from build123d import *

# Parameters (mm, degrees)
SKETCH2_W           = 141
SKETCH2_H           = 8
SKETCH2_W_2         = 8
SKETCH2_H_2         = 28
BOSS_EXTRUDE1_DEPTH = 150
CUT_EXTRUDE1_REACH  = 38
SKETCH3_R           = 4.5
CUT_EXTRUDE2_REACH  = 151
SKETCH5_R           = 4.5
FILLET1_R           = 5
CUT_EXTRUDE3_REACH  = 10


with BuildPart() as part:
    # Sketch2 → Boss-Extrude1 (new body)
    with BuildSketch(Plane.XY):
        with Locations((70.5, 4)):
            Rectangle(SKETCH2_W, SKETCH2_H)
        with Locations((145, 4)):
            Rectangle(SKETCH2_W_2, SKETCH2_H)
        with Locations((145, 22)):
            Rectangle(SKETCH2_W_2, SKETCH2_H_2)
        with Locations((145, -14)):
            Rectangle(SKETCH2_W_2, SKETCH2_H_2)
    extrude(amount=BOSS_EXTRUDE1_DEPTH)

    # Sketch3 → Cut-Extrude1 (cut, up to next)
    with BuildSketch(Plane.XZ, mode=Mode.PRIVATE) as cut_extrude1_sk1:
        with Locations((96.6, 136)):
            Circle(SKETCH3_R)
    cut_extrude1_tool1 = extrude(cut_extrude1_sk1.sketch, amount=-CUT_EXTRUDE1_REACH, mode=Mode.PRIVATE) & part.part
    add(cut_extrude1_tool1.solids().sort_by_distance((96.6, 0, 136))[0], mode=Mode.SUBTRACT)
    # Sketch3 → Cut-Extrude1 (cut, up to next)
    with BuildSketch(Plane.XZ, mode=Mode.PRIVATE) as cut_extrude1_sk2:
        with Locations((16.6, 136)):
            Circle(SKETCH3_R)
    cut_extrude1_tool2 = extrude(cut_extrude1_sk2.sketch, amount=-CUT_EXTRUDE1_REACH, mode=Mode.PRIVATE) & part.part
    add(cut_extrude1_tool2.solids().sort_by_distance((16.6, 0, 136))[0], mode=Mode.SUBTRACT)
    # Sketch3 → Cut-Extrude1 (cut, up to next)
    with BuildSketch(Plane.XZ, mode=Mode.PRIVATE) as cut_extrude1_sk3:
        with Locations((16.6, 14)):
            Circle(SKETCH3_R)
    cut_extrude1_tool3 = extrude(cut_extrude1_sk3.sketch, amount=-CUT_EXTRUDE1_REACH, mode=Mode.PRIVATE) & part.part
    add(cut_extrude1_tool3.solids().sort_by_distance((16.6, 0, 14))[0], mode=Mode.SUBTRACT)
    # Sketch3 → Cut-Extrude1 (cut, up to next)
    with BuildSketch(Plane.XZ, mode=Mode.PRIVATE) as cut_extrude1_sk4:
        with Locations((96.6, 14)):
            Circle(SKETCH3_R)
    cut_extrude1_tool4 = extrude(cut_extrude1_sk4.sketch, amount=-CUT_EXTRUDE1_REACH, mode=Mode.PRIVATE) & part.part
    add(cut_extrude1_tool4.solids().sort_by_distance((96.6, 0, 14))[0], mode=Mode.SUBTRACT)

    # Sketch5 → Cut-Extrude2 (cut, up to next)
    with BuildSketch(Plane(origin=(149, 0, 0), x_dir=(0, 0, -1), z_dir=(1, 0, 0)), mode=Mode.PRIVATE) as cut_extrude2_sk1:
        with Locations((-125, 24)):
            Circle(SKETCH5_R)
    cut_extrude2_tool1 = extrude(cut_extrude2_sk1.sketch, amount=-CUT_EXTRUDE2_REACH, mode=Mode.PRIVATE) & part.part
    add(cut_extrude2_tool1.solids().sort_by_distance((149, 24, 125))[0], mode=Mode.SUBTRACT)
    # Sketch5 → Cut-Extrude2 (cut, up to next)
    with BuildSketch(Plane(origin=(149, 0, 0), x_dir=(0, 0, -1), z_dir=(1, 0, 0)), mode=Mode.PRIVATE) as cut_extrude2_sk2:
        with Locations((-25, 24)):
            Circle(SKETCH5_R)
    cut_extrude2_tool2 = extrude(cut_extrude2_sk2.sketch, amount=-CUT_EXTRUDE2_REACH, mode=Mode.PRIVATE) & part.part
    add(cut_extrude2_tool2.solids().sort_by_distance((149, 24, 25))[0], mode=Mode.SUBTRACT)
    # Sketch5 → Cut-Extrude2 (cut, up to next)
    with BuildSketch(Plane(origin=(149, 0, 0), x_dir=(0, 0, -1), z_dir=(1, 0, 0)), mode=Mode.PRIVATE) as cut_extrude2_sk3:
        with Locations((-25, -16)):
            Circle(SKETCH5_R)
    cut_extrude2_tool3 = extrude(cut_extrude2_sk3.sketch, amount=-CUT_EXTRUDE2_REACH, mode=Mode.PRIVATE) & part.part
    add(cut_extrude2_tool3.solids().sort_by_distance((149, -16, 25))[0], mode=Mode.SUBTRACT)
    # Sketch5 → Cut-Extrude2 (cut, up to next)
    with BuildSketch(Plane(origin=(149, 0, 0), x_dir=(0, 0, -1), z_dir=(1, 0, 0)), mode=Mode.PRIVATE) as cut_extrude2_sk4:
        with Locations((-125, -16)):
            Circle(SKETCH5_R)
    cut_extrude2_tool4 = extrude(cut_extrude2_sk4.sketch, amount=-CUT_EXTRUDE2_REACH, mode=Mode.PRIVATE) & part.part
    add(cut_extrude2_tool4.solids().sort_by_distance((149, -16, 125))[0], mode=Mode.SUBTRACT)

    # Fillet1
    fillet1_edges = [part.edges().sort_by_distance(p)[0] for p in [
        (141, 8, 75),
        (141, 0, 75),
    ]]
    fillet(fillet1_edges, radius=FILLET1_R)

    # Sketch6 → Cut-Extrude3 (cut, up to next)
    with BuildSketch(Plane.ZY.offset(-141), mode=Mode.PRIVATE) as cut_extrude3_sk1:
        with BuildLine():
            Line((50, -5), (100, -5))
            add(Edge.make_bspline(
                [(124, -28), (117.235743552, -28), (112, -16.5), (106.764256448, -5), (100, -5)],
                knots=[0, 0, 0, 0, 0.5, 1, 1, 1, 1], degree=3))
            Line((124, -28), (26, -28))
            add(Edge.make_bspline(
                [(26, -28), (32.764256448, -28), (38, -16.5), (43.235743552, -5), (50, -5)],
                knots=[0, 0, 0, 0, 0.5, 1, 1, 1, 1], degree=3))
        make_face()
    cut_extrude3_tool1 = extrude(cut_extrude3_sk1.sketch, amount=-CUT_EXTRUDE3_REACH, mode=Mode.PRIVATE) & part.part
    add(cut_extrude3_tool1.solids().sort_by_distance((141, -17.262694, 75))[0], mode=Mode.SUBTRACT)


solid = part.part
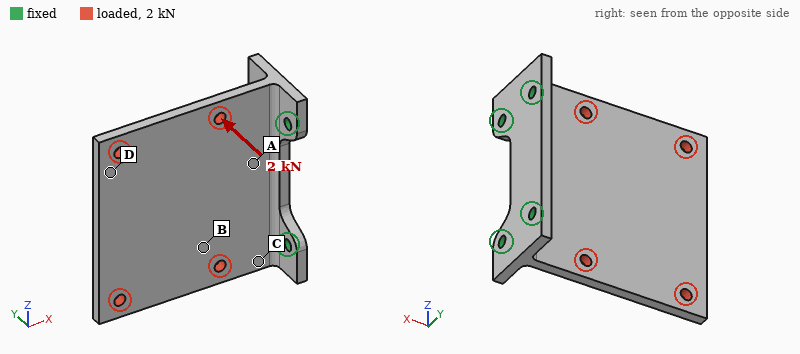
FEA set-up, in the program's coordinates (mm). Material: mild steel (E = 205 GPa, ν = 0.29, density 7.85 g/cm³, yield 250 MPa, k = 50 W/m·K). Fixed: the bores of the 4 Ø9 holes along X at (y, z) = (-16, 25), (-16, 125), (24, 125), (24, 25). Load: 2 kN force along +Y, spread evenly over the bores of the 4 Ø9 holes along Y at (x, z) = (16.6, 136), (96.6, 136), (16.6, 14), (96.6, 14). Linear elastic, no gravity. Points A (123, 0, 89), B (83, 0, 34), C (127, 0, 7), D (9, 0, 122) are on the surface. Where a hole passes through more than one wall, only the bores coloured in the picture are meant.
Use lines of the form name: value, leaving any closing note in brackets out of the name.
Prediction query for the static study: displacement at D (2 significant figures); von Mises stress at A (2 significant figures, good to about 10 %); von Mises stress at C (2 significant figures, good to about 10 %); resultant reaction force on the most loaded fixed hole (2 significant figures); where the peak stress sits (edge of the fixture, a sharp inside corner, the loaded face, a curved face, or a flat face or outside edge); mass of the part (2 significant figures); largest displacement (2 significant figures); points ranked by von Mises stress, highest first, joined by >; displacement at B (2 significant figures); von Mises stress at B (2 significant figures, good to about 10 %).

displacement at D: 0.66 mm
von Mises stress at A: 68 MPa
von Mises stress at C: 93 MPa
resultant reaction force on the most loaded fixed hole: 2.8 kN
where the peak stress sits: a curved face
mass of the part: 1.8 kg
largest displacement: 0.74 mm
points ranked by von Mises stress, highest first, joined by >: C > A > B > D
displacement at B: 0.19 mm
von Mises stress at B: 39 MPa
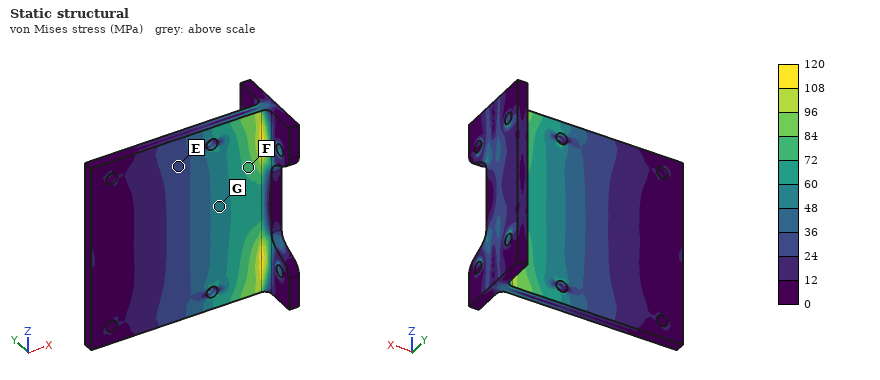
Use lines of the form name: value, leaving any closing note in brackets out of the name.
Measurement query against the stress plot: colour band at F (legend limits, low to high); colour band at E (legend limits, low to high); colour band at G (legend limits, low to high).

colour band at F: 72 to 84 MPa
colour band at E: 24 to 36 MPa
colour band at G: 48 to 60 MPa
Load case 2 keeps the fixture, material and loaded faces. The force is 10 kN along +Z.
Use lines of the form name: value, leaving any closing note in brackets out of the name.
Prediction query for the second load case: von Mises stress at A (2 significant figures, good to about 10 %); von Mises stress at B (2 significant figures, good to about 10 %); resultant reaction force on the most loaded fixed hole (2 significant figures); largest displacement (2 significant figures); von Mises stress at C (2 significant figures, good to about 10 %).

von Mises stress at A: 20 MPa
von Mises stress at B: 13 MPa
resultant reaction force on the most loaded fixed hole: 5.5 kN
largest displacement: 54 µm
von Mises stress at C: 16 MPa
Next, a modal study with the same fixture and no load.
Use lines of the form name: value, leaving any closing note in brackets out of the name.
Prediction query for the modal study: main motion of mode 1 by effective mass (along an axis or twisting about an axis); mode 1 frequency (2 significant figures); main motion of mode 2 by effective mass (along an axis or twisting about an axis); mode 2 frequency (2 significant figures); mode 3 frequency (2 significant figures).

main motion of mode 1 by effective mass: along Y
mode 1 frequency: 320 Hz
main motion of mode 2 by effective mass: twisting about X
mode 2 frequency: 780 Hz
mode 3 frequency: 2000 Hz
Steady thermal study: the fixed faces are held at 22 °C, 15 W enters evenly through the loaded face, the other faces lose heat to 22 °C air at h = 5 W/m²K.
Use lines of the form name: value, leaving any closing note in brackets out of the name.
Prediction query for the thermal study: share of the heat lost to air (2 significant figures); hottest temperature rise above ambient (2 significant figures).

share of the heat lost to air: 23 %
hottest temperature rise above ambient: 24 K
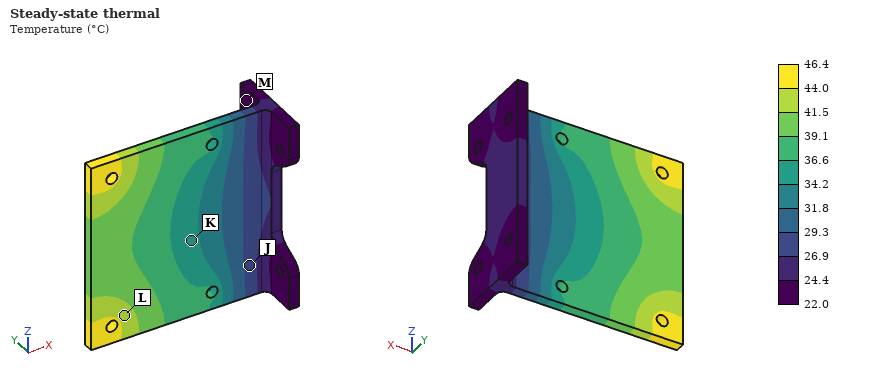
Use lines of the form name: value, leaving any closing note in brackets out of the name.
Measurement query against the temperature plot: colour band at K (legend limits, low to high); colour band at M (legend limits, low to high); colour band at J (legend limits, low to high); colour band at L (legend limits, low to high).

colour band at K: 34.2 to 36.6 °C
colour band at M: 22.0 to 24.4 °C
colour band at J: 26.9 to 29.3 °C
colour band at L: 41.5 to 44.0 °C
